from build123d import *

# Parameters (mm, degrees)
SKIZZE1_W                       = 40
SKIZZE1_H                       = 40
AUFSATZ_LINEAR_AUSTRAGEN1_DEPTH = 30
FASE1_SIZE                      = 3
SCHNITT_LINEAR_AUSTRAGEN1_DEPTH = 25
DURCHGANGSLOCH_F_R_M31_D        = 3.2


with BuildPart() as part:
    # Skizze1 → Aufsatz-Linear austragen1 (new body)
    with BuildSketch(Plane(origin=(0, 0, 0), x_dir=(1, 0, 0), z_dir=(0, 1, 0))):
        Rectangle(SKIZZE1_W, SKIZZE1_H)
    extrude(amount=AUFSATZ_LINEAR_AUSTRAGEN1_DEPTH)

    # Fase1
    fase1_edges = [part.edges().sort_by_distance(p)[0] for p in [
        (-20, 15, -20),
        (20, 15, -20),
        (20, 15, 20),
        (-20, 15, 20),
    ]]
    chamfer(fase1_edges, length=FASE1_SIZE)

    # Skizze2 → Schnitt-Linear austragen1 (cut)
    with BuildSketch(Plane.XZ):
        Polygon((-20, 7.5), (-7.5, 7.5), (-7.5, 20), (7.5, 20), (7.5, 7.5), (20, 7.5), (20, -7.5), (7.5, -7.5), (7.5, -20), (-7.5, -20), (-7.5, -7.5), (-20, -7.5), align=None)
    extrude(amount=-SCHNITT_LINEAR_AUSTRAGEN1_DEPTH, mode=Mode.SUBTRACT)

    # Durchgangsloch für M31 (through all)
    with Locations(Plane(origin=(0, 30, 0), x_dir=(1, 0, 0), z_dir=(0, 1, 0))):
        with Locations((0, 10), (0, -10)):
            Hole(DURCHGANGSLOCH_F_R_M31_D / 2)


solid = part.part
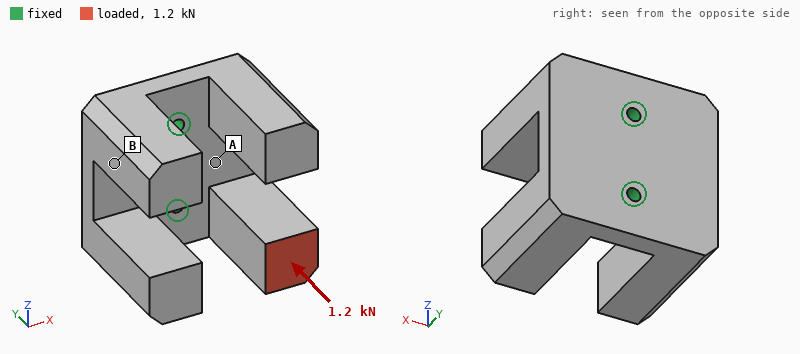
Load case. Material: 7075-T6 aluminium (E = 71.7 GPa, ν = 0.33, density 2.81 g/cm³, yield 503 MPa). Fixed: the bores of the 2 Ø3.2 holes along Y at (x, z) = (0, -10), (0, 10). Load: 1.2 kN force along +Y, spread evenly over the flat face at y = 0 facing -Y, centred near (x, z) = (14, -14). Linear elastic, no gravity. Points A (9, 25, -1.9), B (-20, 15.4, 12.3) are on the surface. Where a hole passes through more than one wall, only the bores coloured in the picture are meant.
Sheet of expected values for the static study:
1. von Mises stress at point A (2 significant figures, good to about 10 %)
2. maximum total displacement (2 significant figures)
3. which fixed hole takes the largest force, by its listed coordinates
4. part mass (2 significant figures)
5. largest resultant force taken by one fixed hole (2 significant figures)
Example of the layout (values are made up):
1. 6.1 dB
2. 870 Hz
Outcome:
1. 54 MPa
2. 0.21 mm
3. (0, -10)
4. 65 g
5. 1.2 kN
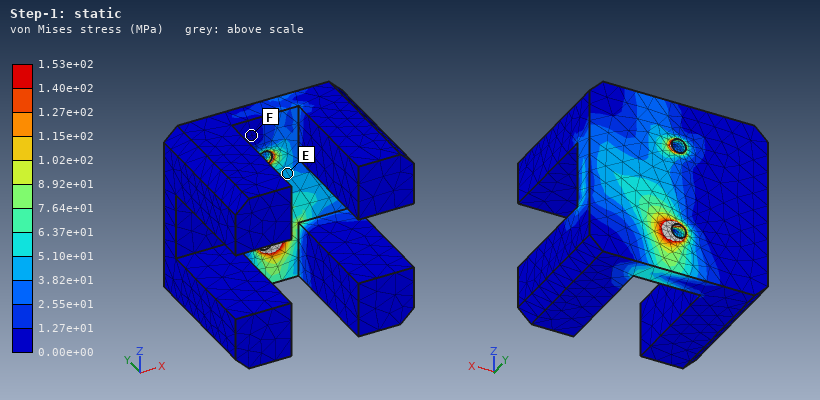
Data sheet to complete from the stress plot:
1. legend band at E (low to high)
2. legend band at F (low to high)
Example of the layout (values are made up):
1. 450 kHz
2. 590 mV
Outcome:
1. 3.82e+01 to 5.10e+01 MPa
2. 0.00e+00 to 1.27e+01 MPa
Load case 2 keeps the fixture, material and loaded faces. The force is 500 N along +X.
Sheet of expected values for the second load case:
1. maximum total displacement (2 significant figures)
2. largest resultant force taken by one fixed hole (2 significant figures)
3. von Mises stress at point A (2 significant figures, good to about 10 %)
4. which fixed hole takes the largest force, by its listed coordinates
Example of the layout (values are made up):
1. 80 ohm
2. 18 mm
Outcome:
1. 0.27 mm
2. 580 N
3. 66 MPa
4. (0, -10)
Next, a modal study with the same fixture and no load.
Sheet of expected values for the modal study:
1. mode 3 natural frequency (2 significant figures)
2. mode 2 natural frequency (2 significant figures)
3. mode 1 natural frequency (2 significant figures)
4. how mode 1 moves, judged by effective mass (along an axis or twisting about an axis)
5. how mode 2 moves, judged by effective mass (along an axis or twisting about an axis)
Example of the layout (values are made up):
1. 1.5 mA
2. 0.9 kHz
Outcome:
1. 3300 Hz
2. 3000 Hz
3. 2500 Hz
4. along X
5. along Y
